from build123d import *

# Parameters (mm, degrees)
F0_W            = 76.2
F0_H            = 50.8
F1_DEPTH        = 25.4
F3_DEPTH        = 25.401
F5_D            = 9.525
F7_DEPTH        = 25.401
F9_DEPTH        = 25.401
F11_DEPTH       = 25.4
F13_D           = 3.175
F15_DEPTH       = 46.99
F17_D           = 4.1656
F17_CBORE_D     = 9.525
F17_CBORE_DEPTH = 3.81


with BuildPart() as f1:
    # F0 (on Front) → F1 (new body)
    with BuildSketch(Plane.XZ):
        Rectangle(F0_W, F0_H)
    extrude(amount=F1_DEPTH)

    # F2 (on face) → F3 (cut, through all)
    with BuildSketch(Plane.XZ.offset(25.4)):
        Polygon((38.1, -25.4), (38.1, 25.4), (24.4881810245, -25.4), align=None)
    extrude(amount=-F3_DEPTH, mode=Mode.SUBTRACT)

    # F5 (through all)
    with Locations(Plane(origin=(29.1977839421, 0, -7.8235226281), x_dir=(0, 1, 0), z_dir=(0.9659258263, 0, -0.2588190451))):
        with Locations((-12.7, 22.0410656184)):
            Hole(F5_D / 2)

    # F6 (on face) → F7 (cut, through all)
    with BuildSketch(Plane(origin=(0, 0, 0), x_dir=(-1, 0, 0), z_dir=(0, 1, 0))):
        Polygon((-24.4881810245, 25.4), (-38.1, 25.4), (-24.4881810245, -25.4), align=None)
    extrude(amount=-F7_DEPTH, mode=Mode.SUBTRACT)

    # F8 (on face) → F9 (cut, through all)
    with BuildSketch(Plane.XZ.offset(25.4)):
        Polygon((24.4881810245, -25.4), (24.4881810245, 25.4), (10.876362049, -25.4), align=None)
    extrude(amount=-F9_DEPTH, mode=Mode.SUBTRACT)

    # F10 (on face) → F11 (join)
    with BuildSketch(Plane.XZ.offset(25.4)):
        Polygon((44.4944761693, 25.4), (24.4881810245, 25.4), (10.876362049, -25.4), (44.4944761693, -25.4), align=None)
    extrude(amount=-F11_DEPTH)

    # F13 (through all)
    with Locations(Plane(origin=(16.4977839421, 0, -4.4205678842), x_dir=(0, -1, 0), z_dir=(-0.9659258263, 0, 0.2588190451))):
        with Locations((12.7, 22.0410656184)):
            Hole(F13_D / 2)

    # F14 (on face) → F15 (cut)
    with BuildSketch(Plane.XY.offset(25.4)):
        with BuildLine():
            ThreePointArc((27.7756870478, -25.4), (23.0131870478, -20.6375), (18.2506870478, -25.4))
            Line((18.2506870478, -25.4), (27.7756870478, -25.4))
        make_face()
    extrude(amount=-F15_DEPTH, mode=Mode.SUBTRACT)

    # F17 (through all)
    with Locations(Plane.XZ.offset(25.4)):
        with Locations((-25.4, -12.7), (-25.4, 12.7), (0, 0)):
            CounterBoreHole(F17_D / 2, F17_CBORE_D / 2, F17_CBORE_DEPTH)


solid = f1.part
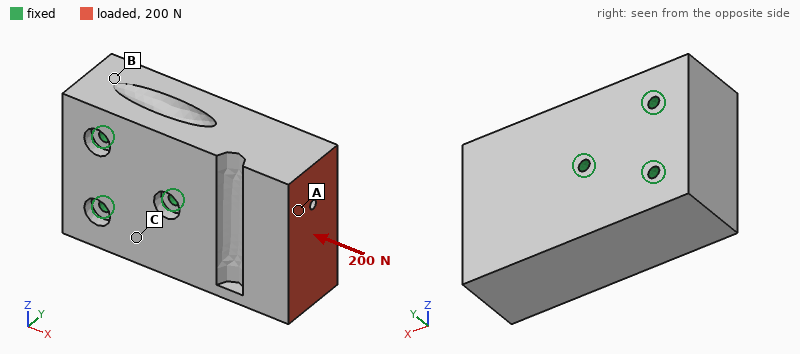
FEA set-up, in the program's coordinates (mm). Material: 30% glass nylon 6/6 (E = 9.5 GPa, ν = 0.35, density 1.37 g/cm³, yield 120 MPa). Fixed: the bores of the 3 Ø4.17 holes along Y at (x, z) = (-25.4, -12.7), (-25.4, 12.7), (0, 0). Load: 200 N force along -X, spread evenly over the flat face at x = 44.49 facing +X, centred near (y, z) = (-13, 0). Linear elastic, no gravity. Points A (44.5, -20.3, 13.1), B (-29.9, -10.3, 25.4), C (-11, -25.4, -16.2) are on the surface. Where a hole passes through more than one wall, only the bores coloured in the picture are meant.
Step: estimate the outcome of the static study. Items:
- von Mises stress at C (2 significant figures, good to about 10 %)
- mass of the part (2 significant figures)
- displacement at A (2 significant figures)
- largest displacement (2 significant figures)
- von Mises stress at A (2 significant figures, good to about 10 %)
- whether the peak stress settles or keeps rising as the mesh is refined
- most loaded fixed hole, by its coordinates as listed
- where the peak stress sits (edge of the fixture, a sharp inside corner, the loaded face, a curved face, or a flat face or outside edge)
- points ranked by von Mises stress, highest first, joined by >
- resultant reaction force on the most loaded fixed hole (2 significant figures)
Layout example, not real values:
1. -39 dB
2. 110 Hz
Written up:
1. 0.10 MPa
2. 140 g
3. 1.5 µm
4. 1.7 µm
5. 0.16 MPa
6. keeps rising
7. (0, 0)
8. edge of the fixture
9. A > C > B
10. 110 N
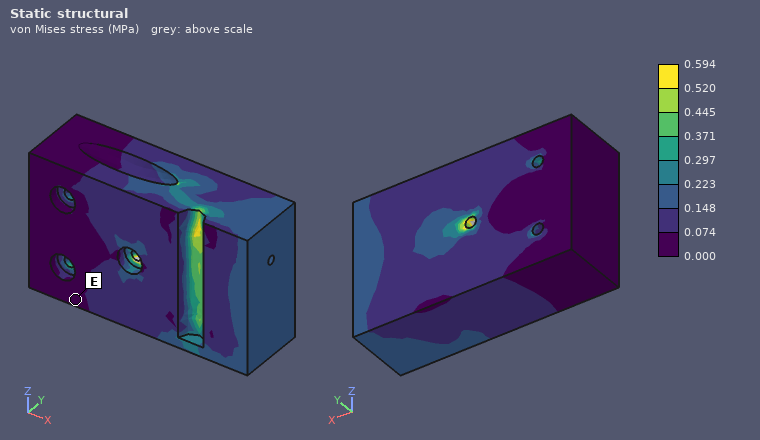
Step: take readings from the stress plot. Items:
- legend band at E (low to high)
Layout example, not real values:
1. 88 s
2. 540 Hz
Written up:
1. 0.000 to 0.074 MPa
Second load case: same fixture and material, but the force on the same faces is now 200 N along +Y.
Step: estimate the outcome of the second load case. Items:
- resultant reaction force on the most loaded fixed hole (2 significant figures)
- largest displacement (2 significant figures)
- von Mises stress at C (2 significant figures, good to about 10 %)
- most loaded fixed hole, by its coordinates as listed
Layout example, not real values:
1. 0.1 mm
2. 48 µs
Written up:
1. 330 N
2. 22 µm
3. 0.82 MPa
4. (0, 0)
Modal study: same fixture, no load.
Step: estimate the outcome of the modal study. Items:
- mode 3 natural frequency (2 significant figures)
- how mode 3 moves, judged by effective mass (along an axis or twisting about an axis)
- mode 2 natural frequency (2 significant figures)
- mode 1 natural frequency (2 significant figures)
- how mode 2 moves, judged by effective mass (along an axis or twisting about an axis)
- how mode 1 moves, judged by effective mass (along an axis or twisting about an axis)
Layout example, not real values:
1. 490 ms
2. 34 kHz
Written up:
1. 4900 Hz
2. twisting about X
3. 4100 Hz
4. 3200 Hz
5. along Z
6. along Y
